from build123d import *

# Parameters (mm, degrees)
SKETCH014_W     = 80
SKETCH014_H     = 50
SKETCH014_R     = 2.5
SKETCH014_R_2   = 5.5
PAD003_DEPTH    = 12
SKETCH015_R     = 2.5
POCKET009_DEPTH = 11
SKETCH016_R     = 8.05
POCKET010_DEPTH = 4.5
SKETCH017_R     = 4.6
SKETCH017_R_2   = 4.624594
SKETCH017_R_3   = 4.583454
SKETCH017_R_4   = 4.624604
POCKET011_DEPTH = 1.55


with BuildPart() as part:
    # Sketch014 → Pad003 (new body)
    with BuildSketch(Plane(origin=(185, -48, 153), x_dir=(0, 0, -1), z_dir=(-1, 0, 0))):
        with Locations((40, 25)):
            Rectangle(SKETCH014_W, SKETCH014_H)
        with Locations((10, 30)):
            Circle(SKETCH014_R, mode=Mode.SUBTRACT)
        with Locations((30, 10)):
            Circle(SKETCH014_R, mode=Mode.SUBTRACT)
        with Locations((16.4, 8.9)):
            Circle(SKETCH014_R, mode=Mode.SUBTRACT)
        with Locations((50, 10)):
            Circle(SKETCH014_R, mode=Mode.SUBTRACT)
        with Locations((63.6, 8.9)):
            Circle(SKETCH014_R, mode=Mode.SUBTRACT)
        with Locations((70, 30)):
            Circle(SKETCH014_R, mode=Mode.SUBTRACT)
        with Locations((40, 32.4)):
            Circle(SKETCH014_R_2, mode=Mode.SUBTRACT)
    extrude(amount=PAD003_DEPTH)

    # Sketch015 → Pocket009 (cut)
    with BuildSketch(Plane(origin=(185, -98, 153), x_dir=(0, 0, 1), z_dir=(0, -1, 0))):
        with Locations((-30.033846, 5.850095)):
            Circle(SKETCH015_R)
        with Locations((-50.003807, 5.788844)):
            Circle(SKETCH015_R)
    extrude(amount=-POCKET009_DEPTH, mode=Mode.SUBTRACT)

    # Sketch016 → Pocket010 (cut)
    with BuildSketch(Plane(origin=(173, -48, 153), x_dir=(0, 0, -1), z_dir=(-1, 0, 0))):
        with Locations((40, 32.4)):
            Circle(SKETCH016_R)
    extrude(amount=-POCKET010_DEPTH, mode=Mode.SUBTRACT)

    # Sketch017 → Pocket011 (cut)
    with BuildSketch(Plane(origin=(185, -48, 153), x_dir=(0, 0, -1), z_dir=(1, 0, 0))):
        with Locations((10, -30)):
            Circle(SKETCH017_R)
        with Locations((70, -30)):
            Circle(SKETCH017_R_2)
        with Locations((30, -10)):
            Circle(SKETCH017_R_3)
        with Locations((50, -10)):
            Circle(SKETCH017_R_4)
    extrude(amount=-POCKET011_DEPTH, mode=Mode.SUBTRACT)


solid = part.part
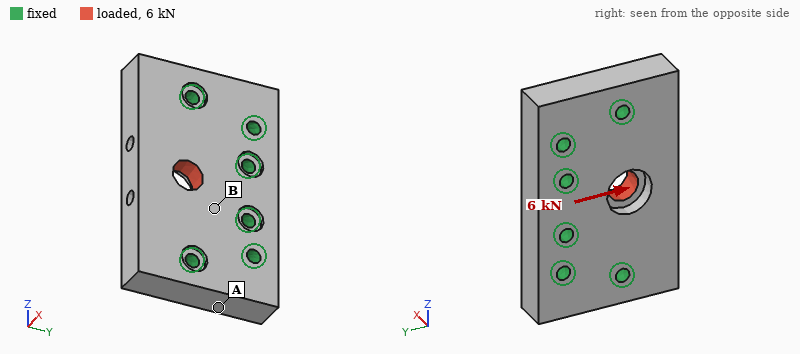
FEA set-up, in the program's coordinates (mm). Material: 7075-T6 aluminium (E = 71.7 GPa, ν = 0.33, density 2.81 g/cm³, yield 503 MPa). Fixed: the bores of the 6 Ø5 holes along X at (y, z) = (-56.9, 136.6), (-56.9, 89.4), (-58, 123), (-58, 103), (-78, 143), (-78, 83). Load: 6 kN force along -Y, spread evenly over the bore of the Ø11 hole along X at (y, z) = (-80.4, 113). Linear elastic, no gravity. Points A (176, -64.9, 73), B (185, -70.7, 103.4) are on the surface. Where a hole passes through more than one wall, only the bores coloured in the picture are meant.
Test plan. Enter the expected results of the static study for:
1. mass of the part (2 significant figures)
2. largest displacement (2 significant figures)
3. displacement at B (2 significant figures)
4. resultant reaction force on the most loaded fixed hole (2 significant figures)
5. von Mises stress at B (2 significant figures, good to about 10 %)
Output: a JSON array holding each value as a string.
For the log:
["120 g", "11 µm", "3.2 µm", "1.9 kN", "18 MPa"]
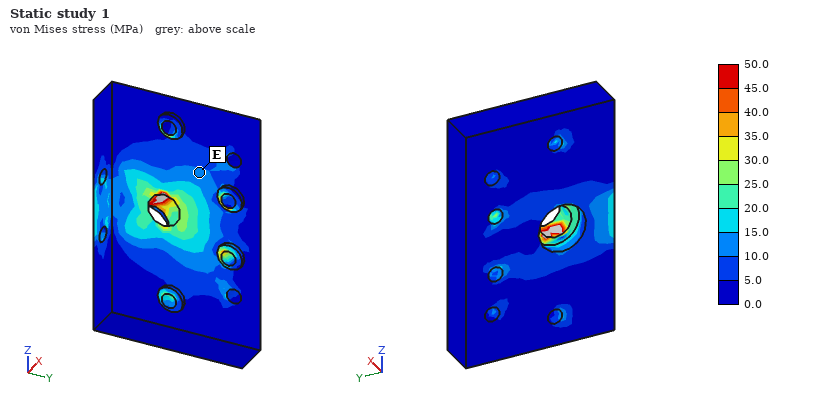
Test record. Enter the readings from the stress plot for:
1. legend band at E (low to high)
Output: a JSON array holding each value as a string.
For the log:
["10.0 to 15.0 MPa"]
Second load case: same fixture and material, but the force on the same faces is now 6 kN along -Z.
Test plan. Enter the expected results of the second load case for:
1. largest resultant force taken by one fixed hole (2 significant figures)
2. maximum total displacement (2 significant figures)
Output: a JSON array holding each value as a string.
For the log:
["2.1 kN", "6.8 µm"]
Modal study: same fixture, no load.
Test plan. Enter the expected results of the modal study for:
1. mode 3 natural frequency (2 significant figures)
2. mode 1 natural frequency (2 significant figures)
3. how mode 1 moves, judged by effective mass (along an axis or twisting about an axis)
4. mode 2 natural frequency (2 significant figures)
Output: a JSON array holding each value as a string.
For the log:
["22 kHz", "11 kHz", "along X", "18 kHz"]
